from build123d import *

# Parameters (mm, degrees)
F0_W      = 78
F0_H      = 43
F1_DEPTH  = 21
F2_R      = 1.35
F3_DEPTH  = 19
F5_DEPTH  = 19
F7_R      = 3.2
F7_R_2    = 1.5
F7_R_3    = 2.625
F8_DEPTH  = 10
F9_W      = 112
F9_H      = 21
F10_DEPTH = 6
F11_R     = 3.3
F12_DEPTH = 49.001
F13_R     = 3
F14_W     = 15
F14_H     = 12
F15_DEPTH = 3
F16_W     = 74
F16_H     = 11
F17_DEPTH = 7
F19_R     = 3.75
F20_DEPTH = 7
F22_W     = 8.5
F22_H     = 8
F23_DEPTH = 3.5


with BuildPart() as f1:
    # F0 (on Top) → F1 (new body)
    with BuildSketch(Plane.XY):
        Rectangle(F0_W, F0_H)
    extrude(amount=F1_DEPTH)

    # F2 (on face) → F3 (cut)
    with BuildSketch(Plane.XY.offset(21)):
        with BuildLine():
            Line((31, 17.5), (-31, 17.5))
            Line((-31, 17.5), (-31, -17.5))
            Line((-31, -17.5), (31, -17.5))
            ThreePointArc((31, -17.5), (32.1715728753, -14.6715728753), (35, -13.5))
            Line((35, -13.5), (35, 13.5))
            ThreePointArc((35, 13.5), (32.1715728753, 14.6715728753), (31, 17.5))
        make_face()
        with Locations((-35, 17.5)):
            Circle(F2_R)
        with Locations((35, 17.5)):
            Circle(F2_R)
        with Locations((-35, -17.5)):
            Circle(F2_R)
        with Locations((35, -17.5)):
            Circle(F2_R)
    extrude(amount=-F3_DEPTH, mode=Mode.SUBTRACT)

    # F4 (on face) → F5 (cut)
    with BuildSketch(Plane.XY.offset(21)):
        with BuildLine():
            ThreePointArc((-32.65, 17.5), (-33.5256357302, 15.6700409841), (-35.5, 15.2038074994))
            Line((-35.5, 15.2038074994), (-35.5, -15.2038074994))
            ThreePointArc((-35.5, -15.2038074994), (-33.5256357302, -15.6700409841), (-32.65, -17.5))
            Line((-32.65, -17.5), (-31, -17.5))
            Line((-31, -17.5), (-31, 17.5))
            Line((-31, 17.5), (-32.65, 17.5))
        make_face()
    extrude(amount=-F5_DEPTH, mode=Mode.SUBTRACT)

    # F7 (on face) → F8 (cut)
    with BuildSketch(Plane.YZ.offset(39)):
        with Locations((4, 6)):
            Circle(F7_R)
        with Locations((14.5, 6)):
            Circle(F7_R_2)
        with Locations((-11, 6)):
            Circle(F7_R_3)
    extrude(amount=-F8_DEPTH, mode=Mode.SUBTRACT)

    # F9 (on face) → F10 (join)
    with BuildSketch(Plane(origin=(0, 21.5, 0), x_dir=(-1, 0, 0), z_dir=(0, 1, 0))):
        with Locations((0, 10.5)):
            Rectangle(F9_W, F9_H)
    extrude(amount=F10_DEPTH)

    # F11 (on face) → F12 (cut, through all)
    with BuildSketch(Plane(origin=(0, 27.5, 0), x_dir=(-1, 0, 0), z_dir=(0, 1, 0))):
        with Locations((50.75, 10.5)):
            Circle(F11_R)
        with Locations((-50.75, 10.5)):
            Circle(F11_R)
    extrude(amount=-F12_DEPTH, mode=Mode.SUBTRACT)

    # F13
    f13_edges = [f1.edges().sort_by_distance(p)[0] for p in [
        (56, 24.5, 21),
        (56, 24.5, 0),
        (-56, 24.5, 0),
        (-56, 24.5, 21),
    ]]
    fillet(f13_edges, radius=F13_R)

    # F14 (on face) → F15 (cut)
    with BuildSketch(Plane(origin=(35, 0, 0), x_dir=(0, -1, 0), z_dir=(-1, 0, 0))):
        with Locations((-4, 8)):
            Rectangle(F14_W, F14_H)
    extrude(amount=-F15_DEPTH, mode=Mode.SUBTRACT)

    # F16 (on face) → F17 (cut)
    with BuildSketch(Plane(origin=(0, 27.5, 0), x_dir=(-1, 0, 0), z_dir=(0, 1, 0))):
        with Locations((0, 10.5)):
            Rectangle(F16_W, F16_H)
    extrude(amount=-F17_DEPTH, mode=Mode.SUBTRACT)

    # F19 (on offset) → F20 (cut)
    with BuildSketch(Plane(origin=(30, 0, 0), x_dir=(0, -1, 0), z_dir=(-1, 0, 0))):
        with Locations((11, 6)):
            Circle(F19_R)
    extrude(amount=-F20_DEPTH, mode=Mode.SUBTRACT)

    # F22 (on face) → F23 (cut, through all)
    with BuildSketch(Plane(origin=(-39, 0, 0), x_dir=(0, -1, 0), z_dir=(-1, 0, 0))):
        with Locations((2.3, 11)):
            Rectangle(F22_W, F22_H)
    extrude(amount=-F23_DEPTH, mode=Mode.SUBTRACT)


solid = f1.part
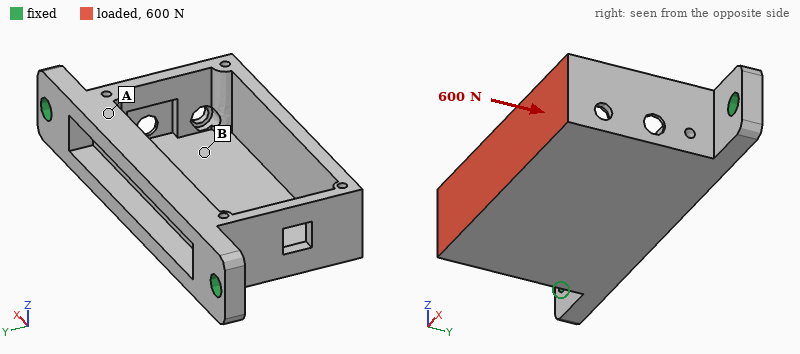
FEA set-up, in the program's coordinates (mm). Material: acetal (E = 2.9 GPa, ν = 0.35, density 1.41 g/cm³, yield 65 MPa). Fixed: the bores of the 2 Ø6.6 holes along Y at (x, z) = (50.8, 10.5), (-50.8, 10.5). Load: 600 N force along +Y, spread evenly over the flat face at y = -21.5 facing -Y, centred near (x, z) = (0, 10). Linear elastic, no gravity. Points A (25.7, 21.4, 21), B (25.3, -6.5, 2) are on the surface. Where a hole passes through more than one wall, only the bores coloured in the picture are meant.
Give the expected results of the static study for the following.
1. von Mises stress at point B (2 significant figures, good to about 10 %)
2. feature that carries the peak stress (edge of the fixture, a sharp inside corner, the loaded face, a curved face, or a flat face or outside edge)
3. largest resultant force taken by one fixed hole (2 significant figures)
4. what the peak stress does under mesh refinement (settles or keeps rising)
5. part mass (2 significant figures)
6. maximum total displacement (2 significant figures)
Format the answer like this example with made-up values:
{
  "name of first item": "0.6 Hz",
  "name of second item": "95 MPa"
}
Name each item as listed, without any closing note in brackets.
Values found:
{
  "von Mises stress at point B": "5.1 MPa",
  "feature that carries the peak stress": "a sharp inside corner",
  "largest resultant force taken by one fixed hole": "340 N",
  "what the peak stress does under mesh refinement": "keeps rising",
  "part mass": "43 g",
  "maximum total displacement": "1.3 mm"
}
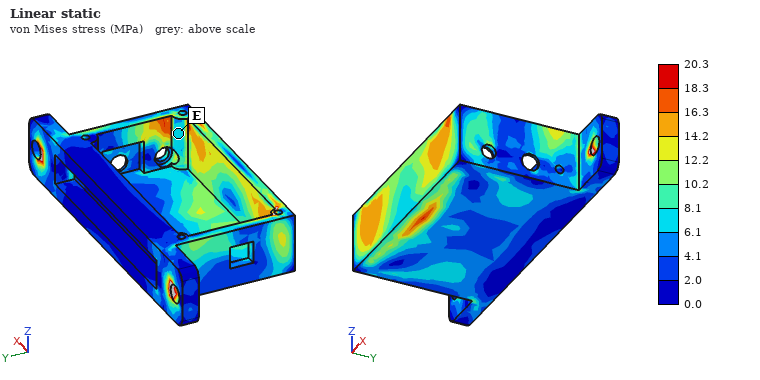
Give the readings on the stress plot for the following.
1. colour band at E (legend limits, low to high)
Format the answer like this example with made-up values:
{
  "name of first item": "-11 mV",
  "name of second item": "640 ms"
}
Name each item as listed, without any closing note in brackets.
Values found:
{
  "colour band at E": "6.1 to 8.1 MPa"
}
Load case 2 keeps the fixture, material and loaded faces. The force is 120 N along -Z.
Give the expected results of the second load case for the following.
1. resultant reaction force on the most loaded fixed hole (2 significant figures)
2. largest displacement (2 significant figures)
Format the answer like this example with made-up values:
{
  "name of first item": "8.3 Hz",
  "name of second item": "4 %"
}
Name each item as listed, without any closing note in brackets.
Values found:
{
  "resultant reaction force on the most loaded fixed hole": "61 N",
  "largest displacement": "1.3 mm"
}
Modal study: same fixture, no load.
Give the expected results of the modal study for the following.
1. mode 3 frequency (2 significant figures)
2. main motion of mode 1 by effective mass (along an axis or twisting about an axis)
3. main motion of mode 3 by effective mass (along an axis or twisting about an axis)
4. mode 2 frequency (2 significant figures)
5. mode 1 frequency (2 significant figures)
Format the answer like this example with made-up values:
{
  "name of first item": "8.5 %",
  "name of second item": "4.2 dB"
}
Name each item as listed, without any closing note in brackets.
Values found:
{
  "mode 3 frequency": "1300 Hz",
  "main motion of mode 1 by effective mass": "along Z",
  "main motion of mode 3 by effective mass": "along Y",
  "mode 2 frequency": "740 Hz",
  "mode 1 frequency": "430 Hz"
}
